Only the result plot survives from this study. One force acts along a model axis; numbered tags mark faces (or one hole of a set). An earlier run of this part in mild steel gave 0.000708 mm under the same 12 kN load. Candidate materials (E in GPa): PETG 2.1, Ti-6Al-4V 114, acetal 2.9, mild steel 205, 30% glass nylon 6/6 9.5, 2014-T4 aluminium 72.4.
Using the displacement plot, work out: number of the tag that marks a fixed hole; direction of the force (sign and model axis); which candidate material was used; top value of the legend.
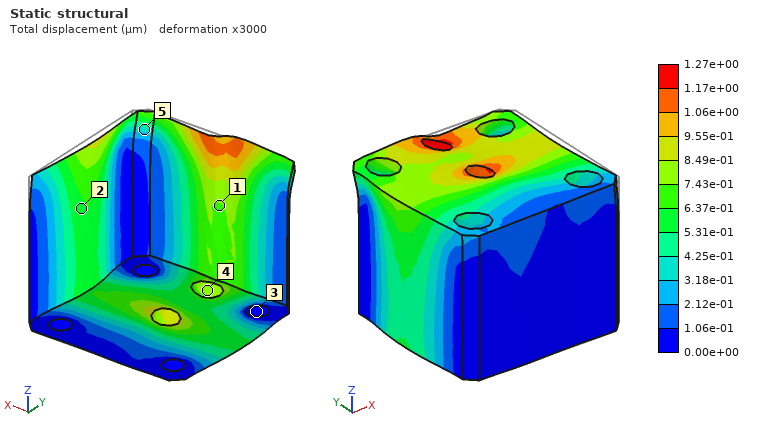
3
-X
Ti-6Al-4V
1.27e+00 µm
